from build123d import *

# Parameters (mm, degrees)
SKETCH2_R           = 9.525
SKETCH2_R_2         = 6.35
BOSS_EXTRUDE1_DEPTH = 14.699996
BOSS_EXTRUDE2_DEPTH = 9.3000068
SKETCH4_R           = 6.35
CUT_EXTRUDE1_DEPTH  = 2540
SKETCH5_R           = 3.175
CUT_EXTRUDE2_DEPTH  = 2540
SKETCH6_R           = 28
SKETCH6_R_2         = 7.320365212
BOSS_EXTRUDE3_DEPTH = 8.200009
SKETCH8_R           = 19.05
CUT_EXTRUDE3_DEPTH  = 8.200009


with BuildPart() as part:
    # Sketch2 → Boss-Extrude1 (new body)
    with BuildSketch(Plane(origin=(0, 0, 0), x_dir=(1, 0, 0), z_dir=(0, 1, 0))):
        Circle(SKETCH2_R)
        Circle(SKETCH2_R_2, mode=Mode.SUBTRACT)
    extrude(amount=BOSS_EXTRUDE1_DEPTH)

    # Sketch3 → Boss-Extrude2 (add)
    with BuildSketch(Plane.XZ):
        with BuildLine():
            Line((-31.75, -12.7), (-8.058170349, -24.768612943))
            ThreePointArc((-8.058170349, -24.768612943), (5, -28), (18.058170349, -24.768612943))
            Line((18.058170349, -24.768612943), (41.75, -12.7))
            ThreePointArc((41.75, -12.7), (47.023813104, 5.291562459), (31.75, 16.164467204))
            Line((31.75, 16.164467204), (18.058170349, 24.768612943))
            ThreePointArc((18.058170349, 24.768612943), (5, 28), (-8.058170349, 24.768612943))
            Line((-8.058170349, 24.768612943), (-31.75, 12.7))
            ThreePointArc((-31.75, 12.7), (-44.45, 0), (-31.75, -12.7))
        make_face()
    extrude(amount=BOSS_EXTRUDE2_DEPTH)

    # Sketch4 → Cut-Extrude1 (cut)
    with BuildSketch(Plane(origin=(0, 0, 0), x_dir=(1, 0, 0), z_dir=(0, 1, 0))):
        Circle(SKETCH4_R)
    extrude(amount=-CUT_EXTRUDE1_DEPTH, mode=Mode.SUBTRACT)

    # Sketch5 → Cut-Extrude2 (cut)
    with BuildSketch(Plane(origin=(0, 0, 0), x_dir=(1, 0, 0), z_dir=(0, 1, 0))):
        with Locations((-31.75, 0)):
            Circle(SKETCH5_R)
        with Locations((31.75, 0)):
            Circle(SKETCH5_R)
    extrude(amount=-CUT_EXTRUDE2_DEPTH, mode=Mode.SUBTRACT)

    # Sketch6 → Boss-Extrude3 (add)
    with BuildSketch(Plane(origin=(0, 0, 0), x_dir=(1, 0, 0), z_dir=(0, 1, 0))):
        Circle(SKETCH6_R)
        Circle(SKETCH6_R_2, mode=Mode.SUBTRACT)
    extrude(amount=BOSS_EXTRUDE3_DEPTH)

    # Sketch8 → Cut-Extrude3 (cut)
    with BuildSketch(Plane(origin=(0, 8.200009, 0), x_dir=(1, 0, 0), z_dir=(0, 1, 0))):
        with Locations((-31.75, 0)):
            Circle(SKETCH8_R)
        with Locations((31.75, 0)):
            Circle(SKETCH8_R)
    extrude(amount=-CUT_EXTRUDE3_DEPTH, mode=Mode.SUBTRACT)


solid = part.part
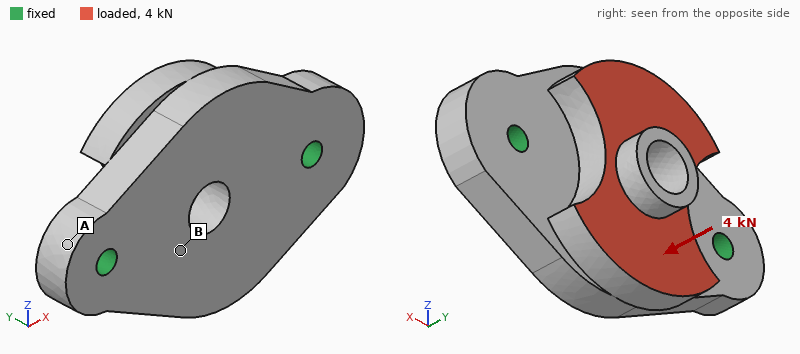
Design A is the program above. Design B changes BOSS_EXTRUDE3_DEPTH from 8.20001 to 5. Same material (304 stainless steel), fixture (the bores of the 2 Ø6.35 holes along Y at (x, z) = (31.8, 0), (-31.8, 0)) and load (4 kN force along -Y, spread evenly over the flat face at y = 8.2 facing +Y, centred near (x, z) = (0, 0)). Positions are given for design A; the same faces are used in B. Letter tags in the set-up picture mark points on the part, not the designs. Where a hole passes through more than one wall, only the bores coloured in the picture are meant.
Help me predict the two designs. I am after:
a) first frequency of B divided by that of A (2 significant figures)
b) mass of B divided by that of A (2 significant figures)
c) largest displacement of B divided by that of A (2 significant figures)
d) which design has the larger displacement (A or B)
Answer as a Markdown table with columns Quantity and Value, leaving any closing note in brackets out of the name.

| Quantity | Value |
|---|---|
| first frequency of B divided by that of A | 1.1 |
| mass of B divided by that of A | 0.90 |
| largest displacement of B divided by that of A | 1.3 |
| which design has the larger displacement | B |
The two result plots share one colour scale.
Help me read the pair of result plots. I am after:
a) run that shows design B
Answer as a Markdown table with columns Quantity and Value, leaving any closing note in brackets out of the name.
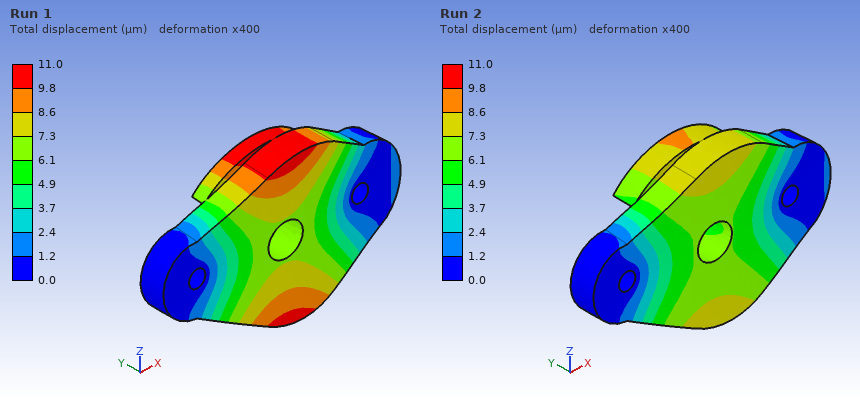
| Quantity | Value |
|---|---|
| run that shows design B | Run 1 |
